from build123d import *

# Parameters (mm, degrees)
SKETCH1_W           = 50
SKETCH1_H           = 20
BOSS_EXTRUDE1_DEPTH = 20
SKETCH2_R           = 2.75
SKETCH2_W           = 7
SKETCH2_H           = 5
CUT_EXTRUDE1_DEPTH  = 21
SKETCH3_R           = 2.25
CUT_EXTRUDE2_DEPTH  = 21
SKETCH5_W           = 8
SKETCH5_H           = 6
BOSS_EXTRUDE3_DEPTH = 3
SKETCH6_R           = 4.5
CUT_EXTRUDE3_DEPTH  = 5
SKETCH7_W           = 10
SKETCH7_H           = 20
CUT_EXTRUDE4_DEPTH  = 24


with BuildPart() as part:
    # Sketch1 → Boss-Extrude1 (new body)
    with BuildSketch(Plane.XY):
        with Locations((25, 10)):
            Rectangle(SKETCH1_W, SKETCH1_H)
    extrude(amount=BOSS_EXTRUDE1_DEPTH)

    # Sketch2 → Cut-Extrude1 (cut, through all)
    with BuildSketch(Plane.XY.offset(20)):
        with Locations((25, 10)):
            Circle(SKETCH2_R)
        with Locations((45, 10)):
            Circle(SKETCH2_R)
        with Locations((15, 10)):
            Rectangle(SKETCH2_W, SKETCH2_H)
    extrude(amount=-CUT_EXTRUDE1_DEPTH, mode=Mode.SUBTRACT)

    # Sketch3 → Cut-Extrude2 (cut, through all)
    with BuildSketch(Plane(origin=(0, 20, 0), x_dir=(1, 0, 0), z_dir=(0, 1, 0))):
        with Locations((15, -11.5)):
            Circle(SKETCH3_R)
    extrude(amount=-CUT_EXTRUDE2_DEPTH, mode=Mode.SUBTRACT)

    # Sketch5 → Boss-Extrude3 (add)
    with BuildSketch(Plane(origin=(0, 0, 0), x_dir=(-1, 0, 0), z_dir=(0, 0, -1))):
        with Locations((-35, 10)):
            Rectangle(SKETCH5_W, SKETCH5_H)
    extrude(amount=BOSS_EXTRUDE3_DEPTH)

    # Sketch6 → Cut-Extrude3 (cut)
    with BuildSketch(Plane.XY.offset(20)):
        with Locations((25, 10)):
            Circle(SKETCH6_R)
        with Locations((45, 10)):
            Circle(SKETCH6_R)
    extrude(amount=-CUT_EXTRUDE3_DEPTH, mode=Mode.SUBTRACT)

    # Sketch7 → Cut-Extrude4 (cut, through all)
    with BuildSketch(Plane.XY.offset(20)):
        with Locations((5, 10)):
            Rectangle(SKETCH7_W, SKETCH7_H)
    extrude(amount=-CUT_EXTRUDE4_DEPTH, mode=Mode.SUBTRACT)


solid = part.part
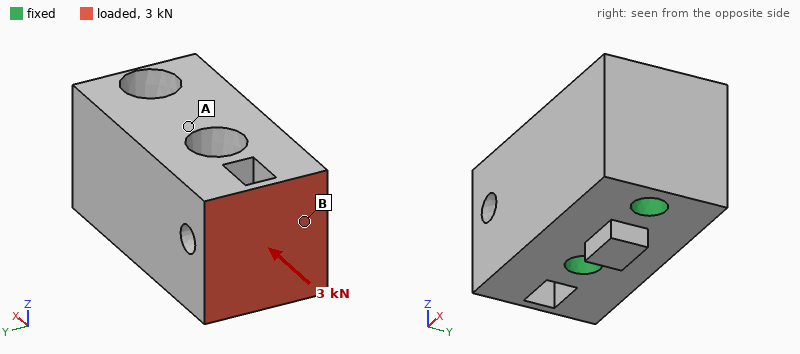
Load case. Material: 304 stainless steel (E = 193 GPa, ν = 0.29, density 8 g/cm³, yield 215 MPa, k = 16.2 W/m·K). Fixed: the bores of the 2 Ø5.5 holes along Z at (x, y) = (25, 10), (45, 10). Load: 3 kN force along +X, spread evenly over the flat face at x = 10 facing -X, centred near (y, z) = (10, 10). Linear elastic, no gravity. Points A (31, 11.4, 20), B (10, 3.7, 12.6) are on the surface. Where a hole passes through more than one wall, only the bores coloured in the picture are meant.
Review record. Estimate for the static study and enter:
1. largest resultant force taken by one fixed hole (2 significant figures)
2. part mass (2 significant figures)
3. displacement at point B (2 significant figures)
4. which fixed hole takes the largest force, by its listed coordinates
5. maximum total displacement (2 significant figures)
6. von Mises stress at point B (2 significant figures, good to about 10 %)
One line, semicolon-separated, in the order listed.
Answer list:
2.4 kN; 110 g; 1.5 µm; (25, 10); 2.7 µm; 11 MPa
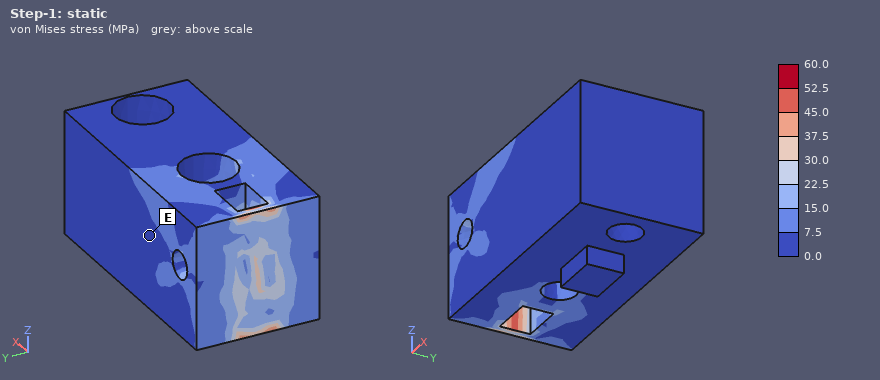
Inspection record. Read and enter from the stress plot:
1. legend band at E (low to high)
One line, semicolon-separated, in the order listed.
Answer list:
0.0 to 7.5 MPa
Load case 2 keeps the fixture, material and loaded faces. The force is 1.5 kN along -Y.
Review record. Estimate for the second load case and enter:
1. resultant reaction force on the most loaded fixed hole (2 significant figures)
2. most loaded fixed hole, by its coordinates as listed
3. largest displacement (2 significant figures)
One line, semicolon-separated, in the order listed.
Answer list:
2.2 kN; (25, 10); 5.6 µm
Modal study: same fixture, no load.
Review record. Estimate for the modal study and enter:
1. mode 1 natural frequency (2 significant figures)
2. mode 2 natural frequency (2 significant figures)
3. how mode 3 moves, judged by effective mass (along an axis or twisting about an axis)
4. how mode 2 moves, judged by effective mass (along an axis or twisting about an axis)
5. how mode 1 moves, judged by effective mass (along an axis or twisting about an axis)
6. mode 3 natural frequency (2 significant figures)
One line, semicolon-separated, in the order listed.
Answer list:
26 kHz; 30 kHz; twisting about X; along Z; along Y; 33 kHz
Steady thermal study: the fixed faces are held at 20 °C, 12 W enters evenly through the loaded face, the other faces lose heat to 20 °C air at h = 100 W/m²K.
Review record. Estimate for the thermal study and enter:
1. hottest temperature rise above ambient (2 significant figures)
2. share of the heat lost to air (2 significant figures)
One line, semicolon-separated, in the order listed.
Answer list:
41 K; 29 %
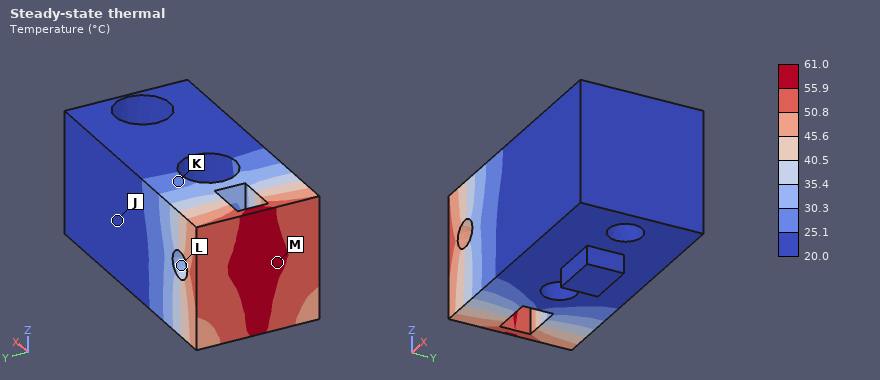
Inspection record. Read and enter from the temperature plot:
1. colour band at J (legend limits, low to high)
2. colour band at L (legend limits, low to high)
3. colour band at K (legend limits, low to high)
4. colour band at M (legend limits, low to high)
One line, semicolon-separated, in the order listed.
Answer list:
20.0 to 25.1 °C; 30.3 to 35.4 °C; 25.1 to 30.3 °C; 55.9 to 61.0 °C
